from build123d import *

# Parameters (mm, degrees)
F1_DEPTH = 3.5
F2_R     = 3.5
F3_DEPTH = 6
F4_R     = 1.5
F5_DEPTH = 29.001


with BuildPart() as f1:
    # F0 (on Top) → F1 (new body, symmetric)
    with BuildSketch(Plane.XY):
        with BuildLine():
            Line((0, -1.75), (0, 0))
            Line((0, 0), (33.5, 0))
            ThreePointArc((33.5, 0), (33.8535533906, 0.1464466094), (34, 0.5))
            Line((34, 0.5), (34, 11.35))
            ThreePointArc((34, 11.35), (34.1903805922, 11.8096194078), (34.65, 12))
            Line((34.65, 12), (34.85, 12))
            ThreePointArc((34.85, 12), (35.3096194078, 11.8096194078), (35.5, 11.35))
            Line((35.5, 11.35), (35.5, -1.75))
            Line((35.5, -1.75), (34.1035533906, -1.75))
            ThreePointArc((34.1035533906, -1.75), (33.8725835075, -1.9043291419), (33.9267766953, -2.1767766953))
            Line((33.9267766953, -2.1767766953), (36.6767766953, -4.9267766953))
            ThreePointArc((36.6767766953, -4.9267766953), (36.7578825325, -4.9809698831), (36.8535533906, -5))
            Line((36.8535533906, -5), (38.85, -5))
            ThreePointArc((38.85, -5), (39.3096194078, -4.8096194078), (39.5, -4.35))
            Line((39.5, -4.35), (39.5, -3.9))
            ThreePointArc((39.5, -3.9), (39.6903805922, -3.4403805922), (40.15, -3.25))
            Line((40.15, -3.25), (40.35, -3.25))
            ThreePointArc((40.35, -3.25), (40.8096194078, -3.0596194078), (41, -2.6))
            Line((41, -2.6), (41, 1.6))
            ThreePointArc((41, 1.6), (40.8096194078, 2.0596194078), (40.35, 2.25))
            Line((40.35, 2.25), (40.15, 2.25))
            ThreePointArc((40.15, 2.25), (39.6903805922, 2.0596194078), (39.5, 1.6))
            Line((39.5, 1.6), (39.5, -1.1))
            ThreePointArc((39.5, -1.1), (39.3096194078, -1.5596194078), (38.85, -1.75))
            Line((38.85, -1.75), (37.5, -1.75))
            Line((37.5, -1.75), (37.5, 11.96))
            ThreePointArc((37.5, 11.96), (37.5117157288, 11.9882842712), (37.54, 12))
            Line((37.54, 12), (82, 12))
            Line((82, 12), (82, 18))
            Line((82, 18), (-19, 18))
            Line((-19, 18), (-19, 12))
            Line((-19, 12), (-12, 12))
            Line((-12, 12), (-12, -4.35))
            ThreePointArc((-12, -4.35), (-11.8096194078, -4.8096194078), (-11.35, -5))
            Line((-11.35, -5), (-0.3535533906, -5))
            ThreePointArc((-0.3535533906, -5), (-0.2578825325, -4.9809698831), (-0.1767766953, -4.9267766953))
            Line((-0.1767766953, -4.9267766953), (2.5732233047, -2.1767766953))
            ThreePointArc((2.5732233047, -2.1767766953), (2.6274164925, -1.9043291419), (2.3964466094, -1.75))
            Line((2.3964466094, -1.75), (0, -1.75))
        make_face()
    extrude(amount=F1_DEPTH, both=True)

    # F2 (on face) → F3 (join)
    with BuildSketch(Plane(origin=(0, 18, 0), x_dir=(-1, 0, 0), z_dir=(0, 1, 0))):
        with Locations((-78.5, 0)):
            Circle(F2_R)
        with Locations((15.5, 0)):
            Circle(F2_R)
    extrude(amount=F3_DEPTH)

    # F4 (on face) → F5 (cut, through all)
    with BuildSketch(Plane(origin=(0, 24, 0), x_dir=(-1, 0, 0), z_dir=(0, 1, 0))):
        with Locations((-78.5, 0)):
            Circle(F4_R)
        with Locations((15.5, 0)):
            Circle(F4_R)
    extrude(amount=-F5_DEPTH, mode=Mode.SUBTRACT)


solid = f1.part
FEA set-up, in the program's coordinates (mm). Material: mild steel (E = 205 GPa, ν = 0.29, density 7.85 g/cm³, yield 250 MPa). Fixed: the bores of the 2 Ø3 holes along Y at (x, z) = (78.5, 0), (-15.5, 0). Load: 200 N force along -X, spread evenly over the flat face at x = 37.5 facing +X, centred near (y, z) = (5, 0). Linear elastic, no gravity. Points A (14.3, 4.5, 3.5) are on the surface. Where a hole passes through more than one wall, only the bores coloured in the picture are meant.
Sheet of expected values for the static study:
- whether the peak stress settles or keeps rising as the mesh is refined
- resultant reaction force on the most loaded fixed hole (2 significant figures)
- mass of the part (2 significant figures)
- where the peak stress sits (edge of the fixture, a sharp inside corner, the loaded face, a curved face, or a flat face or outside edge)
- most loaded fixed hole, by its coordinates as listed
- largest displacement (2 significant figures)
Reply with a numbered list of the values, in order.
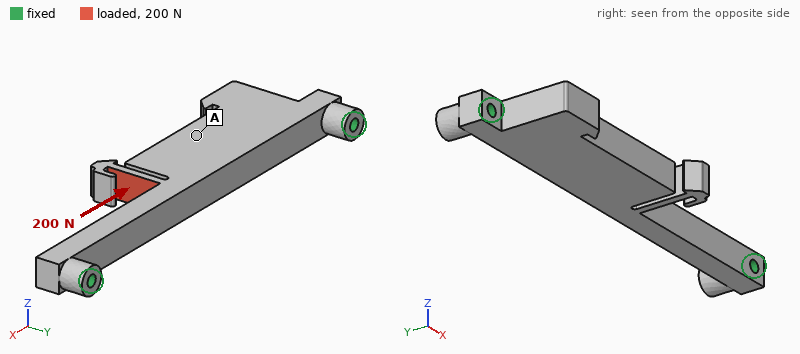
1. keeps rising
2. 130 N
3. 72 g
4. a sharp inside corner
5. (-15.5, 0)
6. 0.11 mm
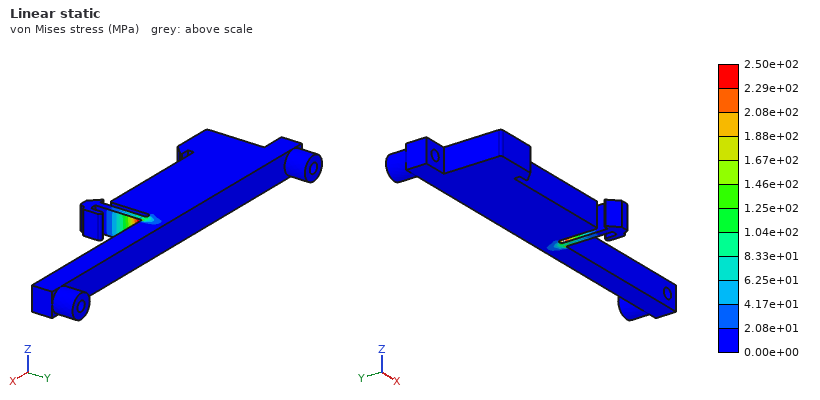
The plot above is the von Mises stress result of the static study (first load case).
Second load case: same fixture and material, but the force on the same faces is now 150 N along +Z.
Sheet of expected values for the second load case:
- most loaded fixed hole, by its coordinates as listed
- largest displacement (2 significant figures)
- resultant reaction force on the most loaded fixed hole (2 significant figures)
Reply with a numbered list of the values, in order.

1. (78.5, 0)
2. 43 µm
3. 86 N
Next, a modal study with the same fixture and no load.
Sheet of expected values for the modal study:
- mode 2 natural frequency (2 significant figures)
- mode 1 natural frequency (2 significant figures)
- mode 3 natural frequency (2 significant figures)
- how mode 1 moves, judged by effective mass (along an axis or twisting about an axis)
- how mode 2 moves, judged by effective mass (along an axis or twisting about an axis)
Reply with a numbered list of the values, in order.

1. 2900 Hz
2. 2700 Hz
3. 3600 Hz
4. along Z
5. along Y
